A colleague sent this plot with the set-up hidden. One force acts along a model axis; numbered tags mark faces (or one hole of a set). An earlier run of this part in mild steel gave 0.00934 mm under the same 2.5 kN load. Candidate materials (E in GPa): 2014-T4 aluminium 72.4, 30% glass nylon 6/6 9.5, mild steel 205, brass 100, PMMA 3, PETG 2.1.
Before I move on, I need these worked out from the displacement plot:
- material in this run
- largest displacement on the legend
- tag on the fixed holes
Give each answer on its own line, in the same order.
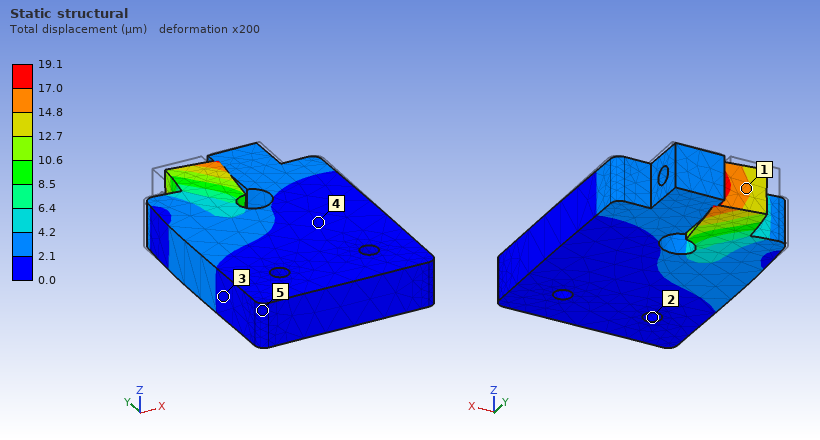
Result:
brass
19.1 µm
2
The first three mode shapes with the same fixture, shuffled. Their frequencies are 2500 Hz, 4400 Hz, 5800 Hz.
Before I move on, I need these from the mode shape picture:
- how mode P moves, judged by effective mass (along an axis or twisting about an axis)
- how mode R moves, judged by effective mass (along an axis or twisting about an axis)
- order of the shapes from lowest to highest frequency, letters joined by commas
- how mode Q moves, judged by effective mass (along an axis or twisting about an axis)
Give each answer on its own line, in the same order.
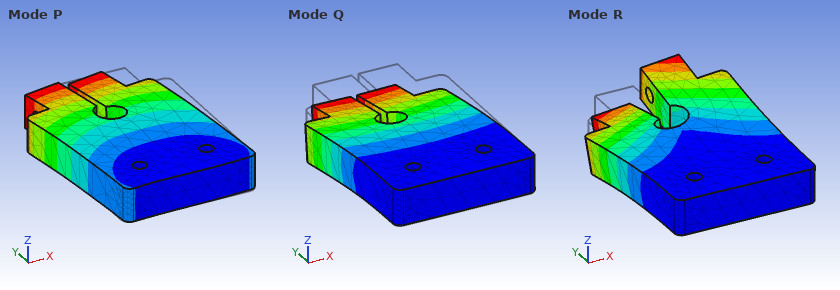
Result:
along X
twisting about Y
Q, R, P
along Z
